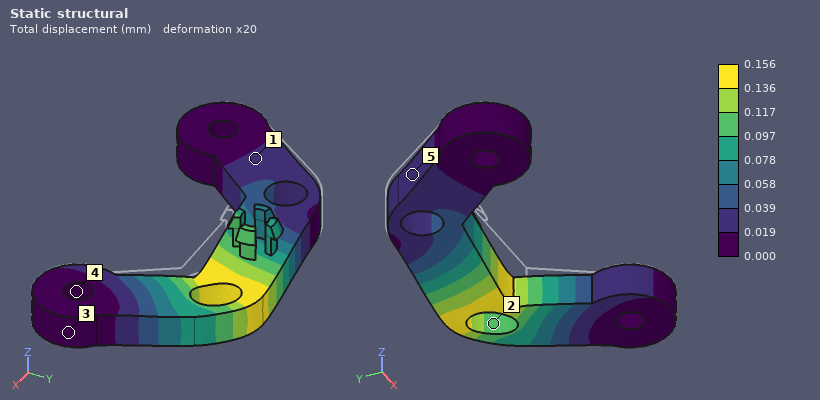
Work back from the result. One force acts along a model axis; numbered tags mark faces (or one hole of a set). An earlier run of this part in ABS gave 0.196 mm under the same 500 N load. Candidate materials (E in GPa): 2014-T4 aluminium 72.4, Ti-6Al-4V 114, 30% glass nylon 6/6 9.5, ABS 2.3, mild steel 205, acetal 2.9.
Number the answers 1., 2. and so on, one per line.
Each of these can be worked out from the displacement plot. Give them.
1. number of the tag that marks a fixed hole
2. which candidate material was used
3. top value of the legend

1. 4
2. acetal
3. 0.156 mm
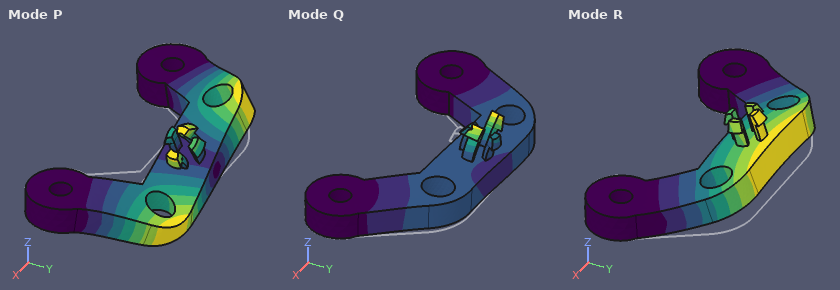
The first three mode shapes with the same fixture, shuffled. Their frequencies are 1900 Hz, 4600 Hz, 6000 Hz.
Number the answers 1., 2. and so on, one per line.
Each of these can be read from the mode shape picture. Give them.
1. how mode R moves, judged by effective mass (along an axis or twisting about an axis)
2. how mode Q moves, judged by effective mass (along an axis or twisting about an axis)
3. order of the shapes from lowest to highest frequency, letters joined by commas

1. along Z
2. along X
3. R, P, Q
